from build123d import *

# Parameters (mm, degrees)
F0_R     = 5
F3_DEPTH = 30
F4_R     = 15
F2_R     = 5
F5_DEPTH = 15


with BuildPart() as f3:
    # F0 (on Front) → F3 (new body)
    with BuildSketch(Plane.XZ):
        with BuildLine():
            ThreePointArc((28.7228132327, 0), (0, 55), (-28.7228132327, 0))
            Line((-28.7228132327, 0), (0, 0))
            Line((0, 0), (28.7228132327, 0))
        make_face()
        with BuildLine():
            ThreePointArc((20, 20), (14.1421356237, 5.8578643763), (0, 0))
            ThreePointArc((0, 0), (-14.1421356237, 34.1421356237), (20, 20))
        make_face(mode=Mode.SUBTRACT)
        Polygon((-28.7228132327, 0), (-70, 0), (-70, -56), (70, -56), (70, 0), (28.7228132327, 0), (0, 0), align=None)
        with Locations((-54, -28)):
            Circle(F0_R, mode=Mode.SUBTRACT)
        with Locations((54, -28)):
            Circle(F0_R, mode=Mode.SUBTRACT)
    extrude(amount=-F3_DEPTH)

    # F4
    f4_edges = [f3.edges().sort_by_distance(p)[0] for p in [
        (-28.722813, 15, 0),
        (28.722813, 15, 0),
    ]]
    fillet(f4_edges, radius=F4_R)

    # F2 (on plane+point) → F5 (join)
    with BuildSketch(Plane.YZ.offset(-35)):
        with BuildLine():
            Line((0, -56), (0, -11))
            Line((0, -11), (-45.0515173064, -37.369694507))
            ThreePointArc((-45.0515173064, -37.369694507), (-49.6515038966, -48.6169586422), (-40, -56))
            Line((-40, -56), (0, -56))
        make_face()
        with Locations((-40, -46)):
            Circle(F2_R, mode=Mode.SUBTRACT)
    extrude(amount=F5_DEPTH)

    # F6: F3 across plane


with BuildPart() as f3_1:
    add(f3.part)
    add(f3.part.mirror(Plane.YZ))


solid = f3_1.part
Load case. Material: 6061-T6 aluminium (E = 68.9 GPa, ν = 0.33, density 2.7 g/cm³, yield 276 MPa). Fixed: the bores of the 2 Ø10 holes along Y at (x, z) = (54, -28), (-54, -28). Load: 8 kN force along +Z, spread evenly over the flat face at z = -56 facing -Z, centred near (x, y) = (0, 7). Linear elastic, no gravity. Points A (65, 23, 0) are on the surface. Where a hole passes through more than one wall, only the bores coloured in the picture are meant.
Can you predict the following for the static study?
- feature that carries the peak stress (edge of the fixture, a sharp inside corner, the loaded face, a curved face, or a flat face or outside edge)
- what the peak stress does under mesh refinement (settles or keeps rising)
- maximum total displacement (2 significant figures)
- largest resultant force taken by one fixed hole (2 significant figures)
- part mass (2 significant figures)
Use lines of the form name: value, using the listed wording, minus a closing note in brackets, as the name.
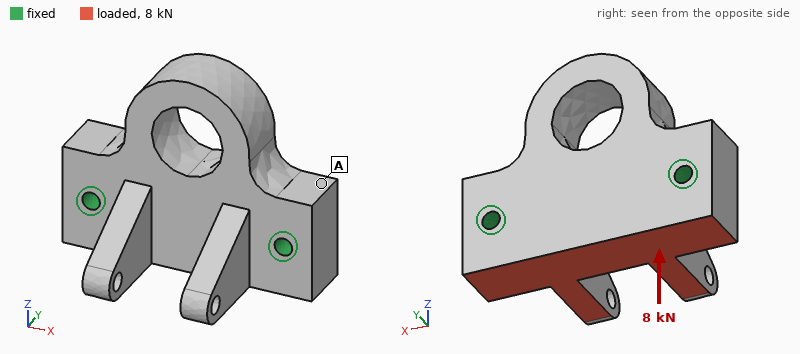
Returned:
feature that carries the peak stress: edge of the fixture
what the peak stress does under mesh refinement: keeps rising
maximum total displacement: 15 µm
largest resultant force taken by one fixed hole: 4.0 kN
part mass: 910 g
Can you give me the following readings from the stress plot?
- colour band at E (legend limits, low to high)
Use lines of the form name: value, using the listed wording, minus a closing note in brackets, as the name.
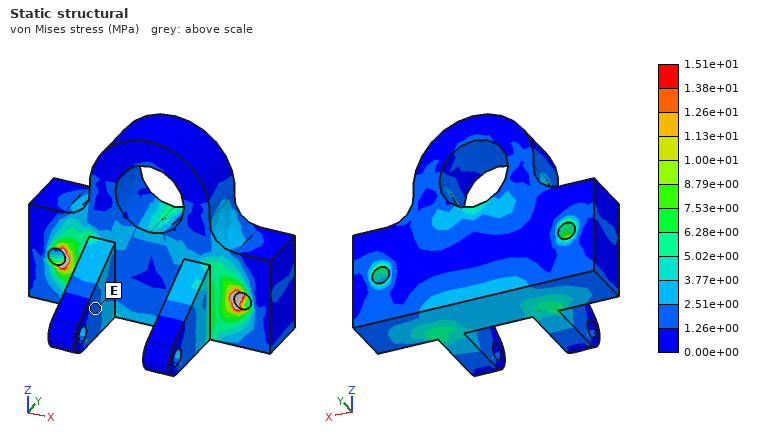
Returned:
colour band at E: 1.26e+00 to 2.51e+00 MPa
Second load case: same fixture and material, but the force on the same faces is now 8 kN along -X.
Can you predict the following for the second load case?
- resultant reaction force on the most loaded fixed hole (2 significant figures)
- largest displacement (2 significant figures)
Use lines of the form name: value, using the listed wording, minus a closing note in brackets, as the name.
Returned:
resultant reaction force on the most loaded fixed hole: 4.5 kN
largest displacement: 28 µm
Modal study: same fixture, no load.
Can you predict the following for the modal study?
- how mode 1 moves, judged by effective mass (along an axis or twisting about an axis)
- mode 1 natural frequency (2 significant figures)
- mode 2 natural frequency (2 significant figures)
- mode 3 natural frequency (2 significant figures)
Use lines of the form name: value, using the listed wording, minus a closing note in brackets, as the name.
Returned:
how mode 1 moves, judged by effective mass: along Y
mode 1 natural frequency: 3300 Hz
mode 2 natural frequency: 5100 Hz
mode 3 natural frequency: 5600 Hz
